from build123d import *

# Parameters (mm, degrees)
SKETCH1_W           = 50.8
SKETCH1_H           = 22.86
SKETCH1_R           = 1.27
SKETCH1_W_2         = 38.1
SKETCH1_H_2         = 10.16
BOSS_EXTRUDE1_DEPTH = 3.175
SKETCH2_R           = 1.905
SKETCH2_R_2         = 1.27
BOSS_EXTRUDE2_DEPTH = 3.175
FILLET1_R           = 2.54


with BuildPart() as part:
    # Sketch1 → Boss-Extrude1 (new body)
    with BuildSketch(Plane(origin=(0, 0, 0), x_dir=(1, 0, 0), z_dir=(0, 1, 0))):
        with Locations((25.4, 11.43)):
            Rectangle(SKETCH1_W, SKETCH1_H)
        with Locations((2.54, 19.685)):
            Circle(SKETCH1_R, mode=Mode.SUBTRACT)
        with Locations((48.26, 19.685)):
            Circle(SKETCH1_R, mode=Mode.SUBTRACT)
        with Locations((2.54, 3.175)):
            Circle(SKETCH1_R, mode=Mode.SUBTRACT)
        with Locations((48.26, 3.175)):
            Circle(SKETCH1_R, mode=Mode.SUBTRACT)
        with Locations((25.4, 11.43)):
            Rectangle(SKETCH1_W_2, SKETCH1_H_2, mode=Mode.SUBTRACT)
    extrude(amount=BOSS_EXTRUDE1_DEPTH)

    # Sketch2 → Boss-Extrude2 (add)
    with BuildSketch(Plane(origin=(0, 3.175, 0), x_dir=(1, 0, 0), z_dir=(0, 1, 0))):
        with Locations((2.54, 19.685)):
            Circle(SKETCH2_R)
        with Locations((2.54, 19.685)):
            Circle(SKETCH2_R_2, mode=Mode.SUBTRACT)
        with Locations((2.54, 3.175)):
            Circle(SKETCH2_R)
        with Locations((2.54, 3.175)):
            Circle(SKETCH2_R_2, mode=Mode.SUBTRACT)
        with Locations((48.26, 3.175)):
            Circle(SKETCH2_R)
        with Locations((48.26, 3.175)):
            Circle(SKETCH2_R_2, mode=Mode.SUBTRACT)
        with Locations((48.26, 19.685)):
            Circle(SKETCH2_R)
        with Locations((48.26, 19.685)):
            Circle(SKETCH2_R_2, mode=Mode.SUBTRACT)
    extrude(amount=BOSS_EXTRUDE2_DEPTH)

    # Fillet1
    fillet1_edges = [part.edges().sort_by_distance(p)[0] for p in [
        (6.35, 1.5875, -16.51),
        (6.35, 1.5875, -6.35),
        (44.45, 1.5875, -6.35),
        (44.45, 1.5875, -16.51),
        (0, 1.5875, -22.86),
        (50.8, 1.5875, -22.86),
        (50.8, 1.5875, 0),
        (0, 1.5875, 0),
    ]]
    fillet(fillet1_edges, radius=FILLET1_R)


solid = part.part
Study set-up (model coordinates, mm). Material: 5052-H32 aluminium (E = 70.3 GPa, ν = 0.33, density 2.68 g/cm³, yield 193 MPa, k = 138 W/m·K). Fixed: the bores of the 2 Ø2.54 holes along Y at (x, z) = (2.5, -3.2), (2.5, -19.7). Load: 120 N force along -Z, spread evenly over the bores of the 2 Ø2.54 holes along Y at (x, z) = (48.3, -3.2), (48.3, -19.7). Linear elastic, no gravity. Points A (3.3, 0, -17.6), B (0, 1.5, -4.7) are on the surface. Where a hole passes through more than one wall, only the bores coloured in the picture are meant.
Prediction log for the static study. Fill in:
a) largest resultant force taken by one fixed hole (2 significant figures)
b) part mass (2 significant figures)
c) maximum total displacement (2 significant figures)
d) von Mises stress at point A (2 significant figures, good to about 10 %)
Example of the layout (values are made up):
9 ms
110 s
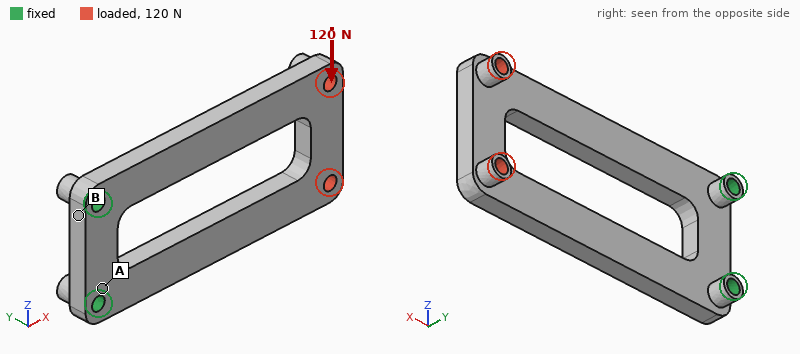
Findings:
270 N
6.6 g
0.12 mm
15 MPa
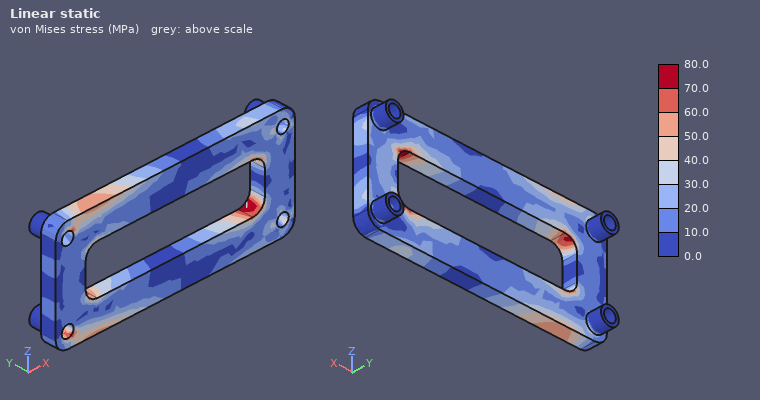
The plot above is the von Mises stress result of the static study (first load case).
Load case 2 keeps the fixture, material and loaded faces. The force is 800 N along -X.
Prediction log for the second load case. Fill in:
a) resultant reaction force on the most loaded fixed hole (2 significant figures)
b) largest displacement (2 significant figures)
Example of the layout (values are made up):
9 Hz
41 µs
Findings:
400 N
0.59 mm
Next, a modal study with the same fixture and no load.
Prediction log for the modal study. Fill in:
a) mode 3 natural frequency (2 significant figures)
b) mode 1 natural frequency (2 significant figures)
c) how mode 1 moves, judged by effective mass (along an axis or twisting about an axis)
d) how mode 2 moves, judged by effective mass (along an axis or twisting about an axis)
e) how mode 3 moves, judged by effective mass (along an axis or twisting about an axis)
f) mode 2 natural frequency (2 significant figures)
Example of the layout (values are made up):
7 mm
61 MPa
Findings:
3500 Hz
1000 Hz
along Y
along Z
twisting about X
3300 Hz
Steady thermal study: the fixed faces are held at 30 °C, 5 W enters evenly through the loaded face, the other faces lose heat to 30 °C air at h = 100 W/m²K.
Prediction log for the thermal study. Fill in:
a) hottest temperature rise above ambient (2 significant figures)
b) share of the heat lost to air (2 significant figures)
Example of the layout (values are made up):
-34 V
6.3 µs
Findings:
26 K
52 %
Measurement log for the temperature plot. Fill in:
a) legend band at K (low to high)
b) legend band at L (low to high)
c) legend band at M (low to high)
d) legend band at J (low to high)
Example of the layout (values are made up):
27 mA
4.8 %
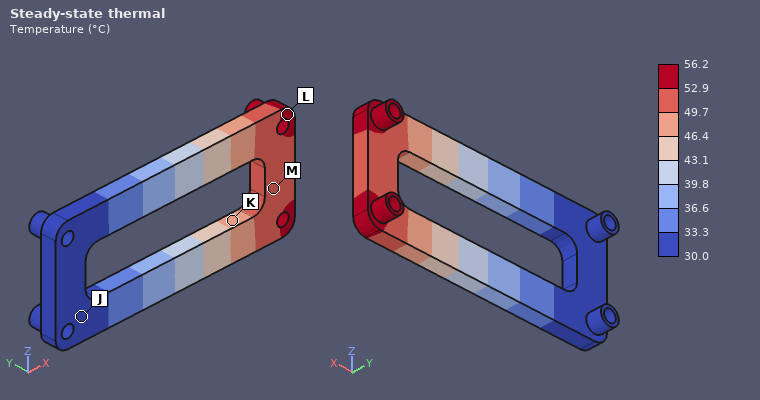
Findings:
46.4 to 49.7 °C
52.9 to 56.2 °C
49.7 to 52.9 °C
30.0 to 33.3 °C
